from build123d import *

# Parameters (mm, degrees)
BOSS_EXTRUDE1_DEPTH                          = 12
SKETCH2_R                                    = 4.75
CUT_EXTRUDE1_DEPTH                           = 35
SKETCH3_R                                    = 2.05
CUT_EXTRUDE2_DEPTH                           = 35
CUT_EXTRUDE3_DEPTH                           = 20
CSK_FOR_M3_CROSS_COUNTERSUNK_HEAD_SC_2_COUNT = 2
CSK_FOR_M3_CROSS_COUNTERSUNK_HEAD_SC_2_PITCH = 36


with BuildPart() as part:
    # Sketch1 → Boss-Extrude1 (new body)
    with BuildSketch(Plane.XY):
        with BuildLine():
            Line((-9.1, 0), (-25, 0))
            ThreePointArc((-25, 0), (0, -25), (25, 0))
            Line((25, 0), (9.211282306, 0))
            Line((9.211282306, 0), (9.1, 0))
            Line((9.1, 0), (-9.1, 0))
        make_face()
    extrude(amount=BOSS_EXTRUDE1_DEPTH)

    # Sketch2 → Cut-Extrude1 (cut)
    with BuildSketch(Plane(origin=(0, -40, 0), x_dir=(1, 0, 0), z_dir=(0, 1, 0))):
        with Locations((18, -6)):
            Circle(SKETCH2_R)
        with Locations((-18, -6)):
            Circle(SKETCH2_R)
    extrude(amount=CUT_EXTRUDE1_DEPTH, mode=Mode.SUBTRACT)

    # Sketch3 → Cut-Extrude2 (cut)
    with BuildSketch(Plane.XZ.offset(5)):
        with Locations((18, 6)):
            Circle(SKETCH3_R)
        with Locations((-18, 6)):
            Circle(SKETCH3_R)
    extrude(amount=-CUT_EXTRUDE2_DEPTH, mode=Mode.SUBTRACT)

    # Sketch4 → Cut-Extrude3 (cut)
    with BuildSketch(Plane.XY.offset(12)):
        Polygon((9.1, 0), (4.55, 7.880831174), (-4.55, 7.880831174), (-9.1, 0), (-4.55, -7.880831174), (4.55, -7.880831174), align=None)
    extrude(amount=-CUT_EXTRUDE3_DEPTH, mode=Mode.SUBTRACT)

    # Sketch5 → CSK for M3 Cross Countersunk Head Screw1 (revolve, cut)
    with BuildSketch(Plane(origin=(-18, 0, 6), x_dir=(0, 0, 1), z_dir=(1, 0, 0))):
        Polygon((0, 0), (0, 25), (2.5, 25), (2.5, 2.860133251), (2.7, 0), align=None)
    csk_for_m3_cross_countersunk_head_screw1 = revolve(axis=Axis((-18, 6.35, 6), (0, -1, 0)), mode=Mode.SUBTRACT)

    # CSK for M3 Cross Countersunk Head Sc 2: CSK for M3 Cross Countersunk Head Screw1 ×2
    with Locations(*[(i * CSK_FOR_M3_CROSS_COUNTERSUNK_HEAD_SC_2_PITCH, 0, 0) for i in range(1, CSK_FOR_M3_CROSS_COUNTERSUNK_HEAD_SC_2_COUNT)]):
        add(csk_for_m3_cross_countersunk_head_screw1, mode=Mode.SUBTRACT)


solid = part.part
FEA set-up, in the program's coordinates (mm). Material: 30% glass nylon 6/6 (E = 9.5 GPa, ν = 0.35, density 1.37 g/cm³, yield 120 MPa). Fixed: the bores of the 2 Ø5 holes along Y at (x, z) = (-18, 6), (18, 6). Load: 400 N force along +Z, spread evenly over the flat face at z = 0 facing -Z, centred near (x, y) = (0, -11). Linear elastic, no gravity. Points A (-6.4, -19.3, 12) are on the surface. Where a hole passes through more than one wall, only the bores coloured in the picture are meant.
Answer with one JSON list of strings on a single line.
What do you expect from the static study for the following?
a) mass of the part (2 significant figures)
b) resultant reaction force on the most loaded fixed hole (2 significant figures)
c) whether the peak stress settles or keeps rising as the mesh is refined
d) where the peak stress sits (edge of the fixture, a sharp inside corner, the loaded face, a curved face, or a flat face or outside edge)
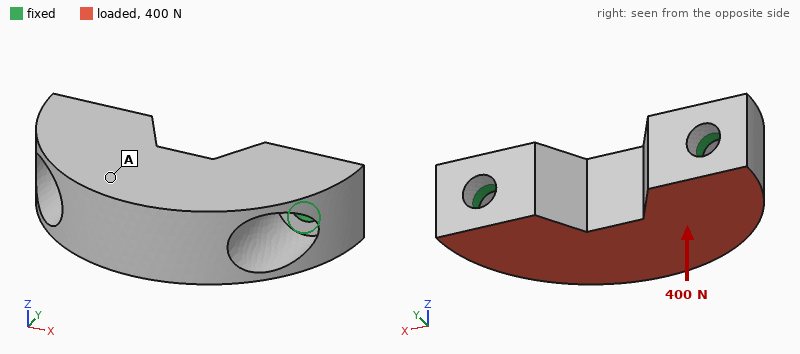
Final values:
["12 g", "200 N", "keeps rising", "edge of the fixture"]
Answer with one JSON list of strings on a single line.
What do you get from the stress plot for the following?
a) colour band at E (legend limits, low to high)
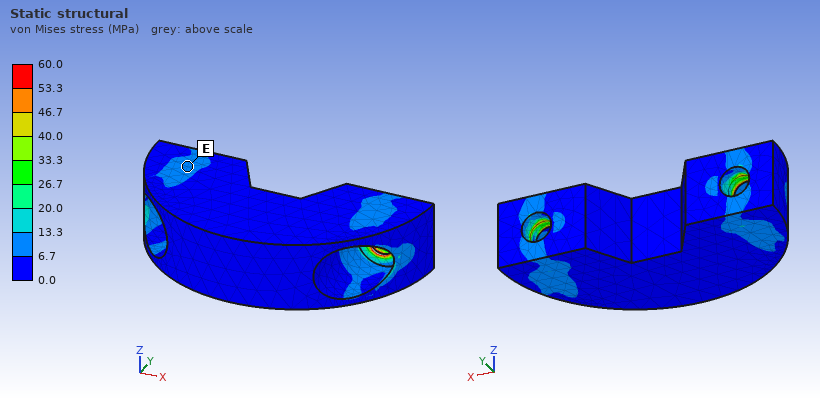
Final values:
["6.7 to 13.3 MPa"]
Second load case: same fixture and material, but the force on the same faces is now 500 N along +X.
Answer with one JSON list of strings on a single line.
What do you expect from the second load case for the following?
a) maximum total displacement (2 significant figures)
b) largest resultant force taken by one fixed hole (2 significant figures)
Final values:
["19 µm", "280 N"]
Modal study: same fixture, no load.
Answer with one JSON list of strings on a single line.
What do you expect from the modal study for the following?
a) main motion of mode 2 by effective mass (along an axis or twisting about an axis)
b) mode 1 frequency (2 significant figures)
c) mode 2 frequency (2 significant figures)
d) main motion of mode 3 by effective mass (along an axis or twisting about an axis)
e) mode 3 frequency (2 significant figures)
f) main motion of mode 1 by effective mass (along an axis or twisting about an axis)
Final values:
["along Y", "3100 Hz", "11 kHz", "twisting about Y", "11 kHz", "along Z"]
